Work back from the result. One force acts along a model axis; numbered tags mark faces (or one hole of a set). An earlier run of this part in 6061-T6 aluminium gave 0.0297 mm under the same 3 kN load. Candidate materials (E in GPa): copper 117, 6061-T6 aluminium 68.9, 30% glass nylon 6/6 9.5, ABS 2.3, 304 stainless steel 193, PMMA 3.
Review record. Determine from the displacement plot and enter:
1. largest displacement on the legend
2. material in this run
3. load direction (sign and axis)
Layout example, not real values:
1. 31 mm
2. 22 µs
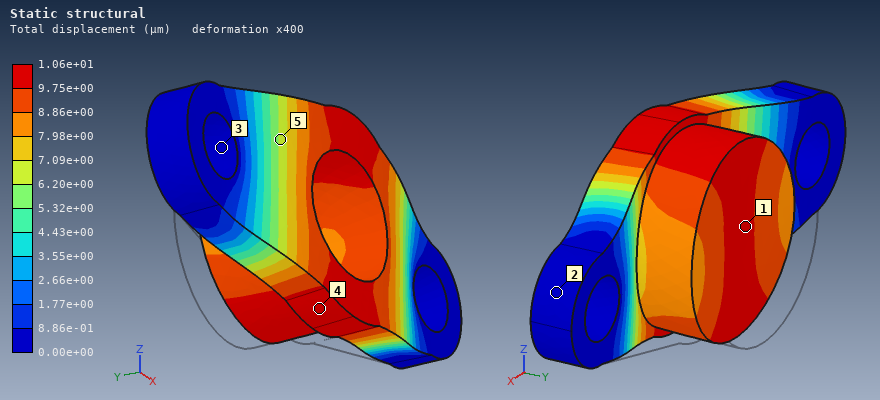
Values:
1. 1.06e+01 µm
2. 304 stainless steel
3. -Y
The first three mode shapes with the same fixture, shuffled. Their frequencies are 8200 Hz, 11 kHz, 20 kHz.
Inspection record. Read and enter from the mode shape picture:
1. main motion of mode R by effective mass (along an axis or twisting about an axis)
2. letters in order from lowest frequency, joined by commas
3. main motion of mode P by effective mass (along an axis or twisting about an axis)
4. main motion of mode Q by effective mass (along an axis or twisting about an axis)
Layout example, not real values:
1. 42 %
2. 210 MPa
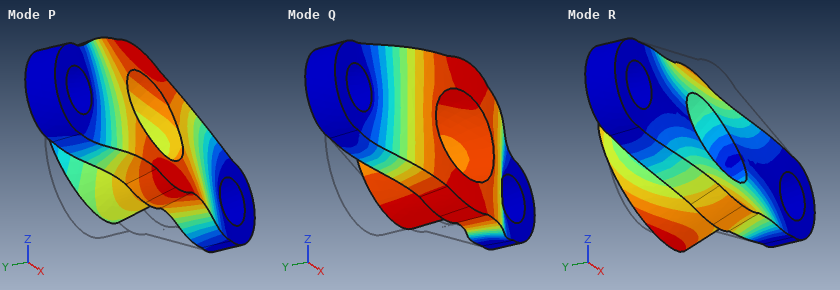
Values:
1. along Z
2. R, Q, P
3. along Z
4. along Y
